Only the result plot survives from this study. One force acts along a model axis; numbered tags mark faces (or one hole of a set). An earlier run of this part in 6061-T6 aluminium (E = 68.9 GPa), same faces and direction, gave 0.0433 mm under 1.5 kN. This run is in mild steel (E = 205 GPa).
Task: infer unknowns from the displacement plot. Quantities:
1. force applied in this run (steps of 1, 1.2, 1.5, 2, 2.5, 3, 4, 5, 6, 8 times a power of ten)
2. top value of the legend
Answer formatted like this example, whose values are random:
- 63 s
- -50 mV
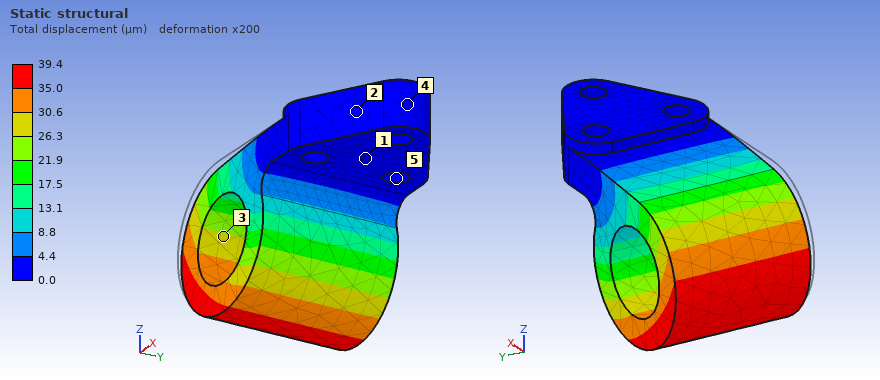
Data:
- 4 kN
- 39.4 µm
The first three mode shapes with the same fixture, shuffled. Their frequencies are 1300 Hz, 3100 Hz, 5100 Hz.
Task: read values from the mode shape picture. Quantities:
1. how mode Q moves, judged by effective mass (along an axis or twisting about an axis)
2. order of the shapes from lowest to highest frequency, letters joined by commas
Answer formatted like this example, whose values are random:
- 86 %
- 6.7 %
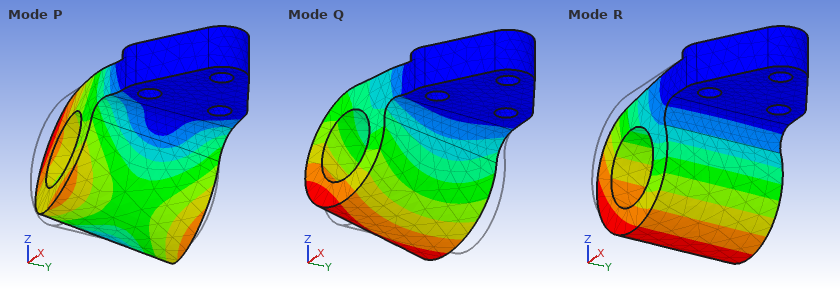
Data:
- along Y
- R, Q, P
